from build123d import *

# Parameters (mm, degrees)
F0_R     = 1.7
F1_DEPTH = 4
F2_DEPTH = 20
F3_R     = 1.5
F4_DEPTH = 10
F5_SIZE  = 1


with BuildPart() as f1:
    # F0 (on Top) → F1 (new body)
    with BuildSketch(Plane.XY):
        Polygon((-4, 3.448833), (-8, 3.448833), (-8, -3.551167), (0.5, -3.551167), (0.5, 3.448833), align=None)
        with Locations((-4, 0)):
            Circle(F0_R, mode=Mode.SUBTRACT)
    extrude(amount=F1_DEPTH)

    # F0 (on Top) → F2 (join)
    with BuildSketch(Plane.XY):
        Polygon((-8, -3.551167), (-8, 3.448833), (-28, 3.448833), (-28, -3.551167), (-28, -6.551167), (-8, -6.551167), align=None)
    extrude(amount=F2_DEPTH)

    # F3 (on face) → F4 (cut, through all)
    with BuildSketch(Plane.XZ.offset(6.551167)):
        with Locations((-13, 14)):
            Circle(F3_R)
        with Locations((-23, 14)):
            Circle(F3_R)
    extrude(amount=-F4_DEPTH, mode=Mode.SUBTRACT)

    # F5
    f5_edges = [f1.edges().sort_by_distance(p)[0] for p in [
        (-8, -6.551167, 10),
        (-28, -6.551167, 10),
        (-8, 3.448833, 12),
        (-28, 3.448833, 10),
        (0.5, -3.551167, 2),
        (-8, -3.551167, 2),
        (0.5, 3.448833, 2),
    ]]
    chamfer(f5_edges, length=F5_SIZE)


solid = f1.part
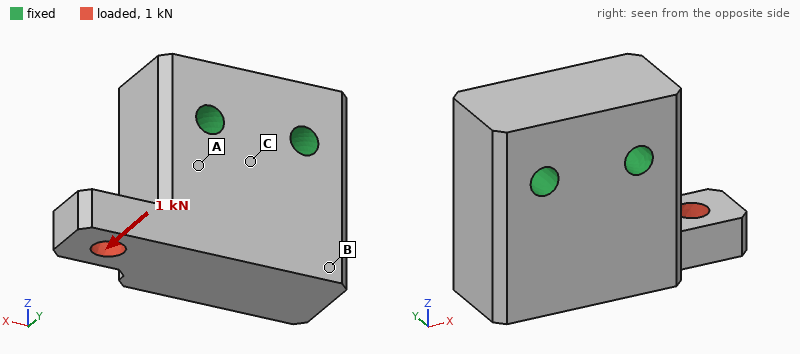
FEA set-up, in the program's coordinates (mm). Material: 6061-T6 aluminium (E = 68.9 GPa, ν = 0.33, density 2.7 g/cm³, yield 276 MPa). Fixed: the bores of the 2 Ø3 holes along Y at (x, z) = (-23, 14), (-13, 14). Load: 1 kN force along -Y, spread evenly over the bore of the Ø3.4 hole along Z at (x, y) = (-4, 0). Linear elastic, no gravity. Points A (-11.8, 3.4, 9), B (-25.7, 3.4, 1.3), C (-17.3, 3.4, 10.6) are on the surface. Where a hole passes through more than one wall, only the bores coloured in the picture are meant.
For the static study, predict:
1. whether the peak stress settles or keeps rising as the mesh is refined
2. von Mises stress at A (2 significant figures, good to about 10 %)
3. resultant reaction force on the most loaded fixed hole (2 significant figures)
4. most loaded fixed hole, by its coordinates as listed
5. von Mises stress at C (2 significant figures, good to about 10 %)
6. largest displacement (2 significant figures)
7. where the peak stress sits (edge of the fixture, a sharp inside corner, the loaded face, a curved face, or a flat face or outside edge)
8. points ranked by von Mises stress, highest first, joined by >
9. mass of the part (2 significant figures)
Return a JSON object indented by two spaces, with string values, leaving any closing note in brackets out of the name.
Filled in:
{
  "whether the peak stress settles or keeps rising as the mesh is refined": "keeps rising",
  "von Mises stress at A": "63 MPa",
  "resultant reaction force on the most loaded fixed hole": "1.2 kN",
  "most loaded fixed hole, by its coordinates as listed": "(-13, 14)",
  "von Mises stress at C": "37 MPa",
  "largest displacement": "71 µm",
  "where the peak stress sits": "a sharp inside corner",
  "points ranked by von Mises stress, highest first, joined by >": "A > C > B",
  "mass of the part": "11 g"
}
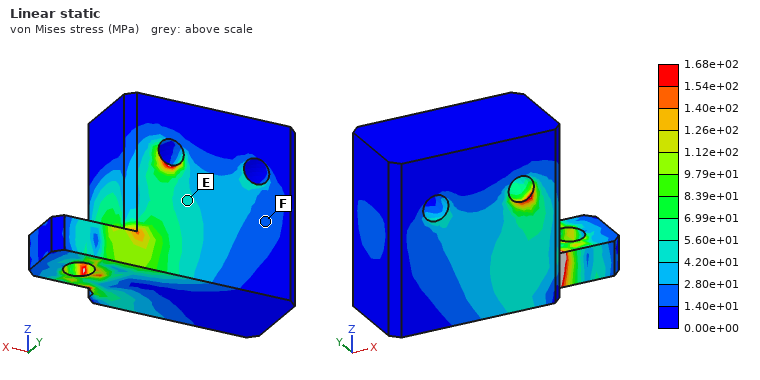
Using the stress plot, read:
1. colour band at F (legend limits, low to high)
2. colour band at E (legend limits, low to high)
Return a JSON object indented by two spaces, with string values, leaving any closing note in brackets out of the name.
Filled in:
{
  "colour band at F": "1.40e+01 to 2.80e+01 MPa",
  "colour band at E": "4.20e+01 to 5.60e+01 MPa"
}
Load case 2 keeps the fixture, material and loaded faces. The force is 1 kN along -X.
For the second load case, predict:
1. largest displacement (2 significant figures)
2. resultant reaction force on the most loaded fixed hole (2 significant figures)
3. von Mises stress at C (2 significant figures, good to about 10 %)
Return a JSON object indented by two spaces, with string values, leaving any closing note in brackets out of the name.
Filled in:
{
  "largest displacement": "18 µm",
  "resultant reaction force on the most loaded fixed hole": "1.1 kN",
  "von Mises stress at C": "17 MPa"
}
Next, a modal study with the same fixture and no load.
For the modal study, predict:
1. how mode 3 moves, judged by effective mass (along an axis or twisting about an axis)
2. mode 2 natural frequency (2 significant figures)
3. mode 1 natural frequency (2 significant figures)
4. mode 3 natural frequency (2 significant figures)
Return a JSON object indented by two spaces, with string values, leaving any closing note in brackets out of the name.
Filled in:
{
  "how mode 3 moves, judged by effective mass": "along Y",
  "mode 2 natural frequency": "26 kHz",
  "mode 1 natural frequency": "25 kHz",
  "mode 3 natural frequency": "34 kHz"
}
